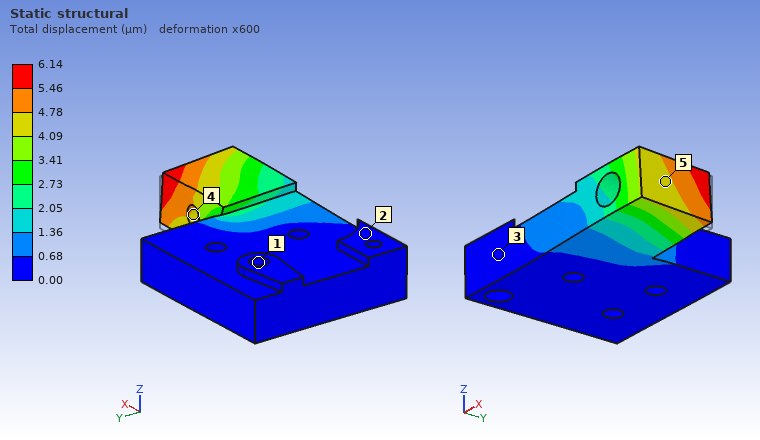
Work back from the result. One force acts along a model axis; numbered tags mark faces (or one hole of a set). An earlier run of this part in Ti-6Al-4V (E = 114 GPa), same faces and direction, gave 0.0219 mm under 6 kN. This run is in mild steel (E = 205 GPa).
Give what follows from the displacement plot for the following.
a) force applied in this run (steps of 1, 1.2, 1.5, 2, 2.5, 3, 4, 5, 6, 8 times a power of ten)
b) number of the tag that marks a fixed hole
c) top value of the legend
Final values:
3 kN
1
6.14 µm
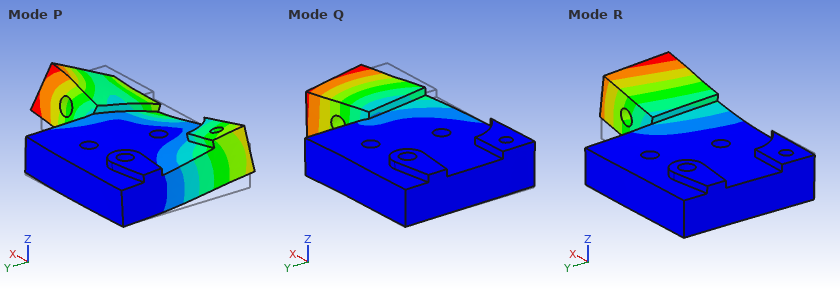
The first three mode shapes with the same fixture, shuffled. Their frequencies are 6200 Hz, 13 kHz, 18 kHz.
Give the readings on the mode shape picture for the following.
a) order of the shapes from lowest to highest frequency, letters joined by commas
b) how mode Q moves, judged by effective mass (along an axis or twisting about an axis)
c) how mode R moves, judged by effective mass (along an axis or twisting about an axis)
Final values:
R, Q, P
along Y
along Z
